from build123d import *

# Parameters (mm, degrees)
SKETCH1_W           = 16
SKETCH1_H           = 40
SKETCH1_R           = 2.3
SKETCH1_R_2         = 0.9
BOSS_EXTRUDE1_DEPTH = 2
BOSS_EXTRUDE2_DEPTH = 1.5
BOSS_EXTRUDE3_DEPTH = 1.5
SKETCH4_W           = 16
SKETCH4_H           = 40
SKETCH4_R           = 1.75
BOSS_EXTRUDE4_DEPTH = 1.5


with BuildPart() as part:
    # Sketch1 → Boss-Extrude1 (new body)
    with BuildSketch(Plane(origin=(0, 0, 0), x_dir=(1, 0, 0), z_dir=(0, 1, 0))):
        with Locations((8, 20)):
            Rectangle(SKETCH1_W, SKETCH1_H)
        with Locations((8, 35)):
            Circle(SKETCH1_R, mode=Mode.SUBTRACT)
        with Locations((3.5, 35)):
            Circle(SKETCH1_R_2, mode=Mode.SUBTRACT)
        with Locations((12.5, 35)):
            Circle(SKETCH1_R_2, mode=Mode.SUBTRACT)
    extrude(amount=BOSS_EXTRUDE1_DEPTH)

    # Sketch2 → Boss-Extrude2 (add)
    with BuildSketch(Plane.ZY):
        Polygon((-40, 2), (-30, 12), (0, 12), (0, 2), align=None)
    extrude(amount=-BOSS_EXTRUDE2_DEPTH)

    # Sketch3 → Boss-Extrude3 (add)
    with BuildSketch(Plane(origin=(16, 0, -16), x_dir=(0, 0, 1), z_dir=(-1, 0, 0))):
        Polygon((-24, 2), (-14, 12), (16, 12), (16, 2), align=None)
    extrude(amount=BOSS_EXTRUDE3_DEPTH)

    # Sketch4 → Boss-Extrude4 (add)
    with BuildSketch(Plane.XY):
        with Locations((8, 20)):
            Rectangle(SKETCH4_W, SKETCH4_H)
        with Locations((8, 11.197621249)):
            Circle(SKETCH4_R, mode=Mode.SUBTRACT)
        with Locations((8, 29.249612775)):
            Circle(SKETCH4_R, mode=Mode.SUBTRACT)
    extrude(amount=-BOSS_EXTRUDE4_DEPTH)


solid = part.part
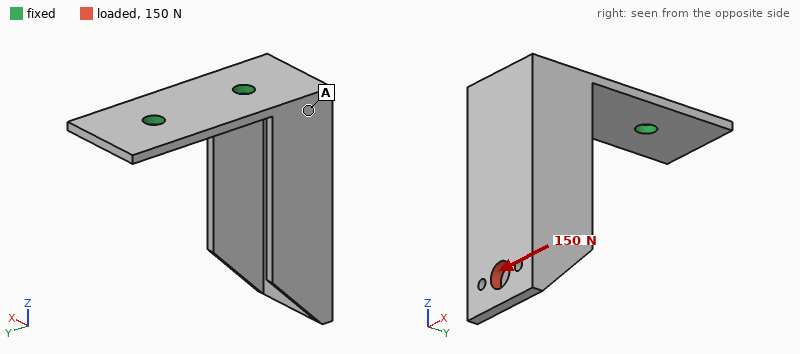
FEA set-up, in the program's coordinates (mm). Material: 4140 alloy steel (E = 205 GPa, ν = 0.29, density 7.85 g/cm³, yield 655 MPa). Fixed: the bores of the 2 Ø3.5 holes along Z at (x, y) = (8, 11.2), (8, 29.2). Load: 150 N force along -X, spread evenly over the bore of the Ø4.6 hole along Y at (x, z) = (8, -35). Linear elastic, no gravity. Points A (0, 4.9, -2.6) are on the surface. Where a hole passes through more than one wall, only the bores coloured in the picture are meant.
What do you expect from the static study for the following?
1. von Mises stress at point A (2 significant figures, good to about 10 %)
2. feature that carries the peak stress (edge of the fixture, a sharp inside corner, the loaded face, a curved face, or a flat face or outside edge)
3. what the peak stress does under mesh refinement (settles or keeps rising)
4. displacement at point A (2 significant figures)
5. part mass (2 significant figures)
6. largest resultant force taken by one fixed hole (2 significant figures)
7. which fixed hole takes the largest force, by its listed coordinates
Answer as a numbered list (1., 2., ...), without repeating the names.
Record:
1. 41 MPa
2. edge of the fixture
3. keeps rising
4. 0.068 mm
5. 25 g
6. 210 N
7. (8, 11.2)
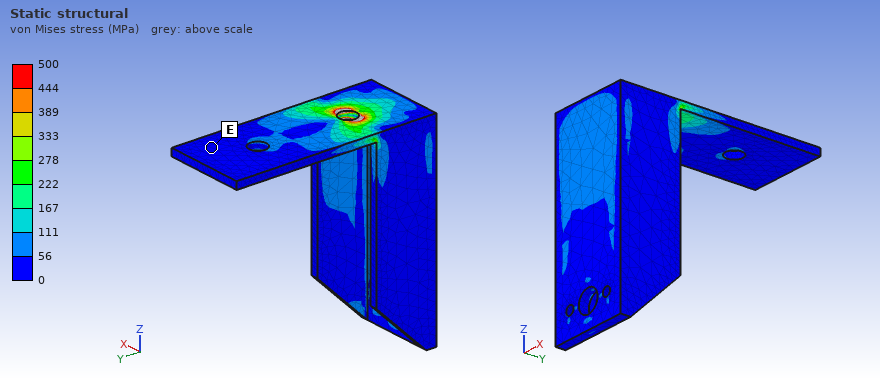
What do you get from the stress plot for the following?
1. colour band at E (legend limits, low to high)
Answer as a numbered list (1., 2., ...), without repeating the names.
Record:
1. 0 to 56 MPa
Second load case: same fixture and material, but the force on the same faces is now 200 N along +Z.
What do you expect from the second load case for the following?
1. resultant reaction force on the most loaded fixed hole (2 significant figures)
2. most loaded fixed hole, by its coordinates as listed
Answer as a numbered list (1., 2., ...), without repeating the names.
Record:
1. 220 N
2. (8, 11.2)
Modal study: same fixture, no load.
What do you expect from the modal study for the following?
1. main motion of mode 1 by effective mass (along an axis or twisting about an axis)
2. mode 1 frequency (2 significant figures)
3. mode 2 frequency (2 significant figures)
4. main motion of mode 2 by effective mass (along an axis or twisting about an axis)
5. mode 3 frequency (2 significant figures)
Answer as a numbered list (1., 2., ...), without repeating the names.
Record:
1. along Y
2. 1100 Hz
3. 1200 Hz
4. along X
5. 5000 Hz
